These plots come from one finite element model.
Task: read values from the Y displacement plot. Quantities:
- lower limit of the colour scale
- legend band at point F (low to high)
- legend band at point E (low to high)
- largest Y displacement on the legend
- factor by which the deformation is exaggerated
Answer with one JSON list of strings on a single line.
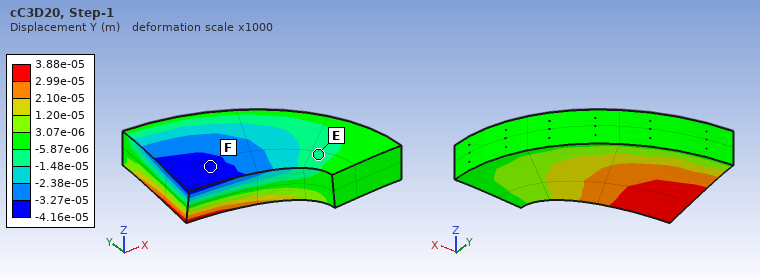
["-4.16e-05 m", "-4.16e-05 to -3.27e-05 m", "-1.48e-05 to -5.87e-06 m", "3.88e-05 m", "1000"]
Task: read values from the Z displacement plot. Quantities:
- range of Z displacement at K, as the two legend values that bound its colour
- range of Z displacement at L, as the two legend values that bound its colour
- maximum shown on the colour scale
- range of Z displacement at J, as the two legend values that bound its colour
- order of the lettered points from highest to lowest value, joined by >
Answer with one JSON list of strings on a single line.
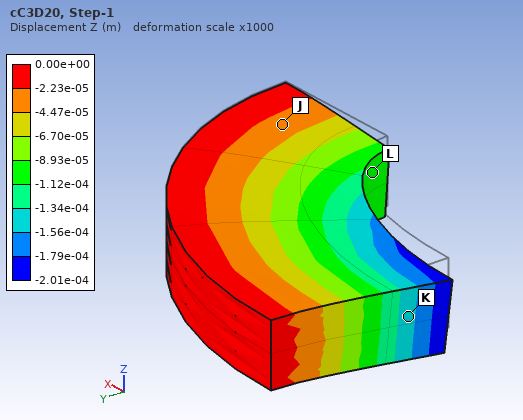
["-1.56e-04 to -1.34e-04 m", "-1.12e-04 to -8.93e-05 m", "0.00e+00 m", "-4.47e-05 to -2.23e-05 m", "J > L > K"]
